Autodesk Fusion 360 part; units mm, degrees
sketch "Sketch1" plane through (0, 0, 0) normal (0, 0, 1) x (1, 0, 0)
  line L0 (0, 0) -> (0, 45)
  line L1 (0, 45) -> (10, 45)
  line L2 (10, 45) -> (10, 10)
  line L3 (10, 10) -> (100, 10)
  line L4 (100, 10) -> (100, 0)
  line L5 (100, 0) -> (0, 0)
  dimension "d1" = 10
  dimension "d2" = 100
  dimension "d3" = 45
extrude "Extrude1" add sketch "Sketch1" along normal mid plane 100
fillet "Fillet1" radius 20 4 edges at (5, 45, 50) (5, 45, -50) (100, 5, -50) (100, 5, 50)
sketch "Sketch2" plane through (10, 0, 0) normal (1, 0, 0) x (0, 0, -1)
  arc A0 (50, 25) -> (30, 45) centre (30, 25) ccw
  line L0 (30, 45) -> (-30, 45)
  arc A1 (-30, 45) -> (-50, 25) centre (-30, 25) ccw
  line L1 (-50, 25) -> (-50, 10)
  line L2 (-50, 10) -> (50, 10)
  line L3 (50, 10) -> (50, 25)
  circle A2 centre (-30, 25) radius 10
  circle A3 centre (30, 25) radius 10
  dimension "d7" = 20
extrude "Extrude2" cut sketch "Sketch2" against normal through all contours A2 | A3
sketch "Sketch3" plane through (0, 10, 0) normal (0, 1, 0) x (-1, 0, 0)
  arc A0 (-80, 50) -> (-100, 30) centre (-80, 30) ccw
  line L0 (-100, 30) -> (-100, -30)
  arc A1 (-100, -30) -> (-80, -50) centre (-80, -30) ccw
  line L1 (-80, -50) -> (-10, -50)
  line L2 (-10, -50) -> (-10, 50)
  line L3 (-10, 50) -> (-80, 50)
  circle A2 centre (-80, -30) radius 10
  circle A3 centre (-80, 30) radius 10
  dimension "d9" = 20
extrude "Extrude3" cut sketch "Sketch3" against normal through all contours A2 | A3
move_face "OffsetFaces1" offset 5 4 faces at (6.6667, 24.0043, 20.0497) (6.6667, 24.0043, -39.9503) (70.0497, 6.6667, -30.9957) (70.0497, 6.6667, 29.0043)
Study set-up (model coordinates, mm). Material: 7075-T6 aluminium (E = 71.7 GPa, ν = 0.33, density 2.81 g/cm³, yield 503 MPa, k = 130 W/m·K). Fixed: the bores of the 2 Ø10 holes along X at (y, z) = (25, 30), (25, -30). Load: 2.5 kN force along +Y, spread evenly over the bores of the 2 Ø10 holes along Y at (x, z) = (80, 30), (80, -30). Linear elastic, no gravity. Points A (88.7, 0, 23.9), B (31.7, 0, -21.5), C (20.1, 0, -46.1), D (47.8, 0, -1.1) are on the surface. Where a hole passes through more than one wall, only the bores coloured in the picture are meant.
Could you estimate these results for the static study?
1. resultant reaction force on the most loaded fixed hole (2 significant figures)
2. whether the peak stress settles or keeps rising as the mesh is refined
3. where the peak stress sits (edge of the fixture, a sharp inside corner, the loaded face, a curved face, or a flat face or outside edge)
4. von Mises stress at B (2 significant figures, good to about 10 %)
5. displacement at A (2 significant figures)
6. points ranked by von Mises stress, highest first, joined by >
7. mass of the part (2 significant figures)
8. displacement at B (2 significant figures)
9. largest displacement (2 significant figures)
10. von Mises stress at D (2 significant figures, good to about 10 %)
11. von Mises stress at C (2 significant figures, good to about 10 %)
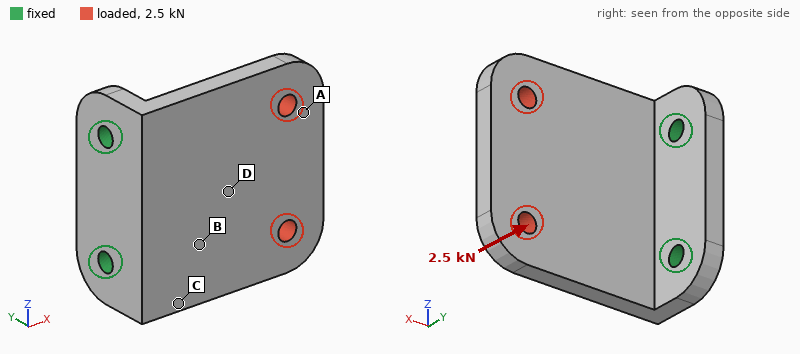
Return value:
1.3 kN
keeps rising
edge of the fixture
65 MPa
1.1 mm
C > B > D > A
360 g
0.26 mm
1.3 mm
41 MPa
91 MPa
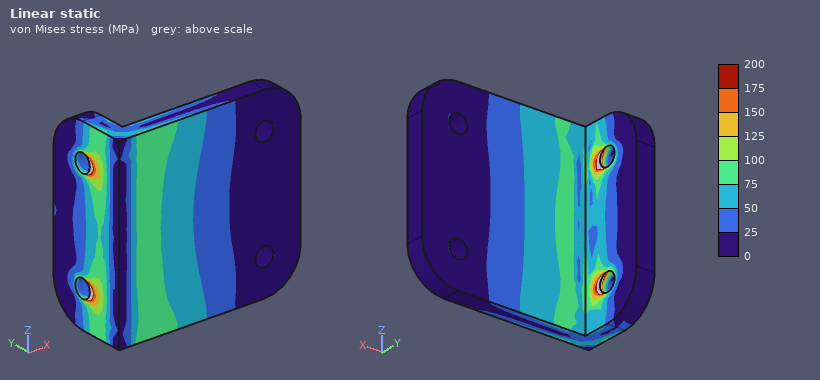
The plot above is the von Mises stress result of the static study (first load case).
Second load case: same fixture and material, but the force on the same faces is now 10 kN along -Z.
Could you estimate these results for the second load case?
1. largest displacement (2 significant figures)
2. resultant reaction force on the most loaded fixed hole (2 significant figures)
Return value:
0.38 mm
13 kN
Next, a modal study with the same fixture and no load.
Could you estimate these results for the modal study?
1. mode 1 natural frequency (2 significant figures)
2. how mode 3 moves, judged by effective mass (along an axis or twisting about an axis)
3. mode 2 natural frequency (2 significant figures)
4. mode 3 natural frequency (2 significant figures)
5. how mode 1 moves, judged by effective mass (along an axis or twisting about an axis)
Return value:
730 Hz
along Z
1900 Hz
2800 Hz
along Y
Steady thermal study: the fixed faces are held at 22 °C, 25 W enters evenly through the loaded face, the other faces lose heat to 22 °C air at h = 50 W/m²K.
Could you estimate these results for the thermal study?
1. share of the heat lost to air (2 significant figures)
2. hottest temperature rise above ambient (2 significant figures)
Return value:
38 %
15 K
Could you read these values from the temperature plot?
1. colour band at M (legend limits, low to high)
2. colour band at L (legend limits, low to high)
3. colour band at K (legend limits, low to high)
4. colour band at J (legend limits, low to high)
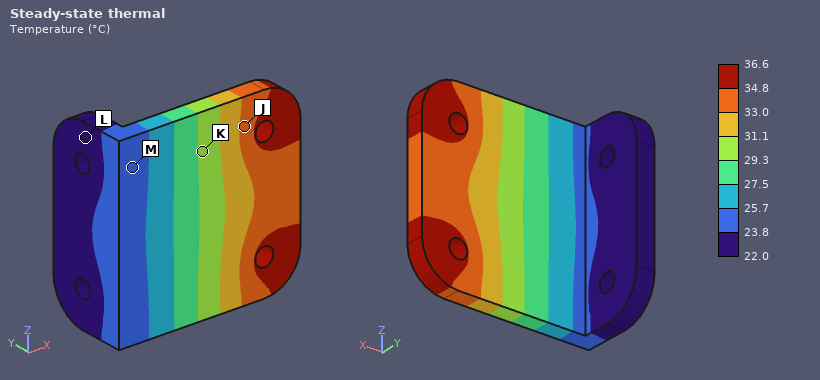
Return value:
23.8 to 25.7 °C
22.0 to 23.8 °C
29.3 to 31.1 °C
33.0 to 34.8 °C
